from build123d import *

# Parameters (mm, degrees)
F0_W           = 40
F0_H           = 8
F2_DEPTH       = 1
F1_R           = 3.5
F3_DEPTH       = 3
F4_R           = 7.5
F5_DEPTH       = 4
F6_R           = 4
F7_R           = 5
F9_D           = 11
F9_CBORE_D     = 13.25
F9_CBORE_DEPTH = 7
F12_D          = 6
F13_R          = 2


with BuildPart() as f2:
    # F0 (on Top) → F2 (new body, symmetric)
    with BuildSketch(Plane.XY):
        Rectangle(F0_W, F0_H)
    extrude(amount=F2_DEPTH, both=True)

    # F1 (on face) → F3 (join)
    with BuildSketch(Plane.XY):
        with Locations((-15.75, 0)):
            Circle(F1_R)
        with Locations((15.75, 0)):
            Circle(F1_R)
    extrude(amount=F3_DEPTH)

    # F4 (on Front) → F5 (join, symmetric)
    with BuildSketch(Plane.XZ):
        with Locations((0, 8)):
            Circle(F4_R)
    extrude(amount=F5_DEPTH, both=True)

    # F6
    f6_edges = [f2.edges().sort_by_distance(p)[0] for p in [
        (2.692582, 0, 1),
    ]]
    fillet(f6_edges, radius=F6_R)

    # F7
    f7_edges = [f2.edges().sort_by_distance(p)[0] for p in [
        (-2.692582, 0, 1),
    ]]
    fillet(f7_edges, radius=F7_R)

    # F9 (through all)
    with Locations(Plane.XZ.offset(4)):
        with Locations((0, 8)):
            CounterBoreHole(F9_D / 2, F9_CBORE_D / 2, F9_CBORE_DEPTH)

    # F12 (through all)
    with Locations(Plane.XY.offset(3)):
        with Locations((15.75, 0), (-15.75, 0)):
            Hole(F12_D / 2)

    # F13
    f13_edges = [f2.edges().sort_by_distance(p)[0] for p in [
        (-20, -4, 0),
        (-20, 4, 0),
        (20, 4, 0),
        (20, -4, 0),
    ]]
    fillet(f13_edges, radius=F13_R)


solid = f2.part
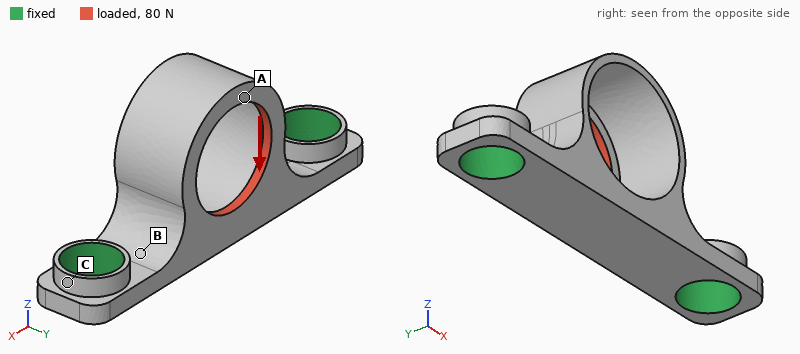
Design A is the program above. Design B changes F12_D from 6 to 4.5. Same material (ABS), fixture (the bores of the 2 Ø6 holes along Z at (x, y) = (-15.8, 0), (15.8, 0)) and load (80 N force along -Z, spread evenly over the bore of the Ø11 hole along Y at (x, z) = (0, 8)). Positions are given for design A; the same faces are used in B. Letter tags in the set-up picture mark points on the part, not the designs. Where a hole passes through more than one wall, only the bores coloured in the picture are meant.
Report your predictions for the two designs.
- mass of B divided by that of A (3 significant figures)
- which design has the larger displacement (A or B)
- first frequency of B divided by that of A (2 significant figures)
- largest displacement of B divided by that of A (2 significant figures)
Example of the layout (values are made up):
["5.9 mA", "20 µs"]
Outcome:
["1.09", "B", "0.94", "1.1"]
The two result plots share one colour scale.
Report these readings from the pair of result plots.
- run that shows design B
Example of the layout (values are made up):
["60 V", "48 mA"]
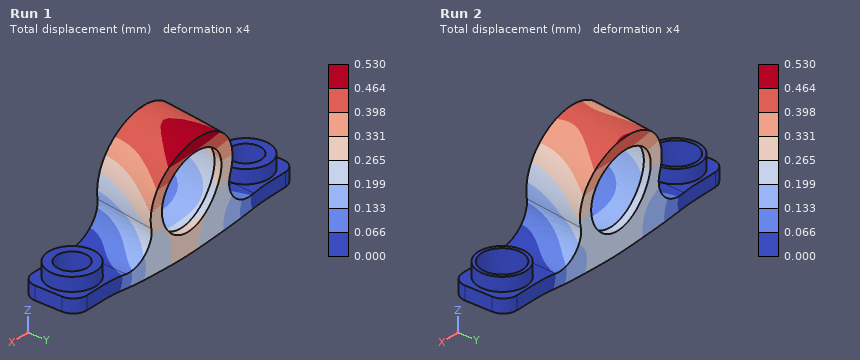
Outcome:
["Run 1"]
